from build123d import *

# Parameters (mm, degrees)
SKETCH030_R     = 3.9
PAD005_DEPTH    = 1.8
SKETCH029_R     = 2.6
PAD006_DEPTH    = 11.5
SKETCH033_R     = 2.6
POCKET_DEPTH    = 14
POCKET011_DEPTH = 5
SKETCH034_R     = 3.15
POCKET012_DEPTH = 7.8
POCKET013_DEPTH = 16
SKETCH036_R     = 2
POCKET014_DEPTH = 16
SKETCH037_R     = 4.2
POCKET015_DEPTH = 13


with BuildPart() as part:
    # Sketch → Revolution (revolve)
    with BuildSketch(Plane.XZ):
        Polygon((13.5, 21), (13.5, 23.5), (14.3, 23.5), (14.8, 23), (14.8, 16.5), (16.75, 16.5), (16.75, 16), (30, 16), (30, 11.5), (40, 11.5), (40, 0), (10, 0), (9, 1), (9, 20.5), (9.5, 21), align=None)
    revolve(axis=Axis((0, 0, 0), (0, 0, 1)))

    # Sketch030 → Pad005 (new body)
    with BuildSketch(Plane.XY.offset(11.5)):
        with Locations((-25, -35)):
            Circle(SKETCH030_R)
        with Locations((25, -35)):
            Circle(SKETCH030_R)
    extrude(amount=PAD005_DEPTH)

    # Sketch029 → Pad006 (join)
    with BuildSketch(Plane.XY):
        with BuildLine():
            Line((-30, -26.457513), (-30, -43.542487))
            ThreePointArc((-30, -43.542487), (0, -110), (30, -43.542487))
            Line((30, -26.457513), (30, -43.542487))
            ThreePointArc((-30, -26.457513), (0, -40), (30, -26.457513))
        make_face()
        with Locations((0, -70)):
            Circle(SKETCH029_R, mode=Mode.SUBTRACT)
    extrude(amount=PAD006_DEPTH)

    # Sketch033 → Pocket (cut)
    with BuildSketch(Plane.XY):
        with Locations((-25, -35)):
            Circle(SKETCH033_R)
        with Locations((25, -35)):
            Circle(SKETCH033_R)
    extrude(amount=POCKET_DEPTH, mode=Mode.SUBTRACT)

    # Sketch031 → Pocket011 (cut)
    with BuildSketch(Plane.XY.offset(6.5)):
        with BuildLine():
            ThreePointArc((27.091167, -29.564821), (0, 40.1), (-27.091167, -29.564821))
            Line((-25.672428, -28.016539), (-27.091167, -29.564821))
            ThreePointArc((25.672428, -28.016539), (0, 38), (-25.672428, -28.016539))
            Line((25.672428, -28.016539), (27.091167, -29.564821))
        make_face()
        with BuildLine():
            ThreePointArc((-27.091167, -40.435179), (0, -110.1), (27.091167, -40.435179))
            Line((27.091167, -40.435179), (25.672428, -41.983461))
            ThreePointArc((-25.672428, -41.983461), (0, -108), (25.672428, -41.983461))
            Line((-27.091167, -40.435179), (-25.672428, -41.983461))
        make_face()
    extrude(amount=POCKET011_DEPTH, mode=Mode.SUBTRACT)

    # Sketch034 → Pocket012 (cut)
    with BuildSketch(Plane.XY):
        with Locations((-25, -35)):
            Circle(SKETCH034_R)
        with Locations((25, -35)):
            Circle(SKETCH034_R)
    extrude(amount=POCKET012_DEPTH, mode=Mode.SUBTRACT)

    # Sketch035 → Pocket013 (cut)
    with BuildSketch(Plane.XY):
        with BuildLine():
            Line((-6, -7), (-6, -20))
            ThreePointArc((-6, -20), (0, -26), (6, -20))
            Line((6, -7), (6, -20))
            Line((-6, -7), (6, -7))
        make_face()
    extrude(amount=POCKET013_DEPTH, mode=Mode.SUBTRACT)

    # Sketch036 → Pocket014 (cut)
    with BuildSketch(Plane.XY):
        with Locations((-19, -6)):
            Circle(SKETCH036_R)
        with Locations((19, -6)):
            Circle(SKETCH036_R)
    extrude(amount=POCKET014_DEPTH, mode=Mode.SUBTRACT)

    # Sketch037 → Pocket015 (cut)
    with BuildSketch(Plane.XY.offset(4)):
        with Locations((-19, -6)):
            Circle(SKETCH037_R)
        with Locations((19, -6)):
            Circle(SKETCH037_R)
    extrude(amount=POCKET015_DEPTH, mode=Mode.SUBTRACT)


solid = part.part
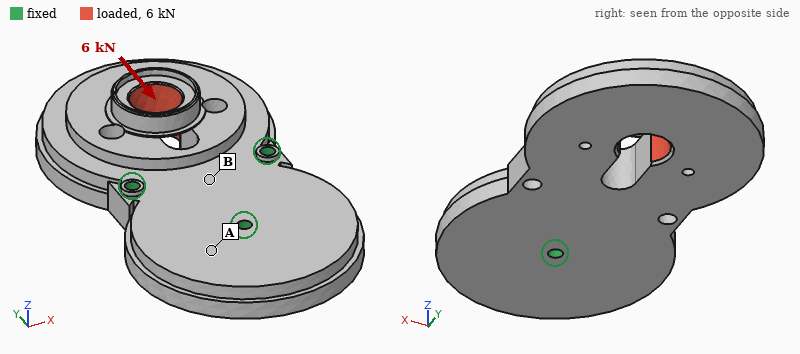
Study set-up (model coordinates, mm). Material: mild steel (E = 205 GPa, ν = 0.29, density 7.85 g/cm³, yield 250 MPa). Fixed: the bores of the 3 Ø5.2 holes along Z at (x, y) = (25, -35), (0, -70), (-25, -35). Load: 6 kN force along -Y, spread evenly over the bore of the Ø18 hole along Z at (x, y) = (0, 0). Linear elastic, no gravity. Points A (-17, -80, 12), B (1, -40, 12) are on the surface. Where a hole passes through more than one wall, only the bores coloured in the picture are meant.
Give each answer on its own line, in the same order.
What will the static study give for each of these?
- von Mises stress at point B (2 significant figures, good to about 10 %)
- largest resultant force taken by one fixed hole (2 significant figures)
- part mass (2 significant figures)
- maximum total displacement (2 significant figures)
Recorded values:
16 MPa
2.4 kN
910 g
34 µm
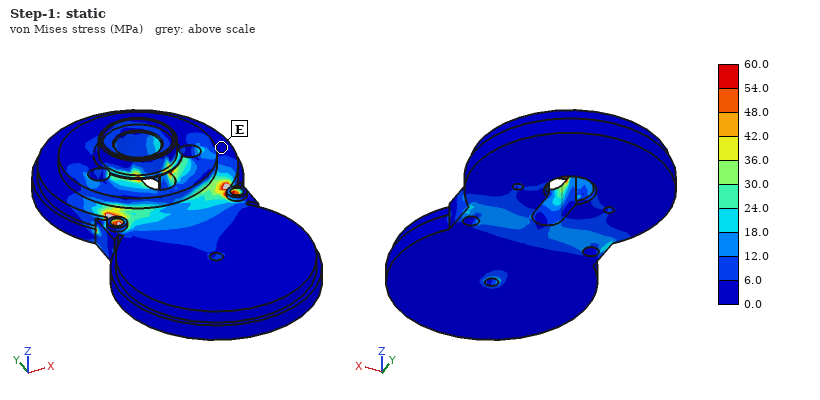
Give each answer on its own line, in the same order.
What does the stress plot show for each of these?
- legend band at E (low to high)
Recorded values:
0.0 to 6.0 MPa
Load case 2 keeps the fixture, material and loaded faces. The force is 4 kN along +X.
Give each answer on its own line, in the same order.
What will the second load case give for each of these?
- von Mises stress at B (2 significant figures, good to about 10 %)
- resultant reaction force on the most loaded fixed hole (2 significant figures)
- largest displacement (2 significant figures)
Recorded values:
12 MPa
3.4 kN
16 µm
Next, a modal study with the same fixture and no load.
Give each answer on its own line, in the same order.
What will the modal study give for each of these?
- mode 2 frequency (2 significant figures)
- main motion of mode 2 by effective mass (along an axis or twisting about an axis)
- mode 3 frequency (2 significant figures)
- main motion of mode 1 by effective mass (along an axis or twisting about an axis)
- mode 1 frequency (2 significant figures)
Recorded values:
4200 Hz
along X
4400 Hz
along Z
1400 Hz
